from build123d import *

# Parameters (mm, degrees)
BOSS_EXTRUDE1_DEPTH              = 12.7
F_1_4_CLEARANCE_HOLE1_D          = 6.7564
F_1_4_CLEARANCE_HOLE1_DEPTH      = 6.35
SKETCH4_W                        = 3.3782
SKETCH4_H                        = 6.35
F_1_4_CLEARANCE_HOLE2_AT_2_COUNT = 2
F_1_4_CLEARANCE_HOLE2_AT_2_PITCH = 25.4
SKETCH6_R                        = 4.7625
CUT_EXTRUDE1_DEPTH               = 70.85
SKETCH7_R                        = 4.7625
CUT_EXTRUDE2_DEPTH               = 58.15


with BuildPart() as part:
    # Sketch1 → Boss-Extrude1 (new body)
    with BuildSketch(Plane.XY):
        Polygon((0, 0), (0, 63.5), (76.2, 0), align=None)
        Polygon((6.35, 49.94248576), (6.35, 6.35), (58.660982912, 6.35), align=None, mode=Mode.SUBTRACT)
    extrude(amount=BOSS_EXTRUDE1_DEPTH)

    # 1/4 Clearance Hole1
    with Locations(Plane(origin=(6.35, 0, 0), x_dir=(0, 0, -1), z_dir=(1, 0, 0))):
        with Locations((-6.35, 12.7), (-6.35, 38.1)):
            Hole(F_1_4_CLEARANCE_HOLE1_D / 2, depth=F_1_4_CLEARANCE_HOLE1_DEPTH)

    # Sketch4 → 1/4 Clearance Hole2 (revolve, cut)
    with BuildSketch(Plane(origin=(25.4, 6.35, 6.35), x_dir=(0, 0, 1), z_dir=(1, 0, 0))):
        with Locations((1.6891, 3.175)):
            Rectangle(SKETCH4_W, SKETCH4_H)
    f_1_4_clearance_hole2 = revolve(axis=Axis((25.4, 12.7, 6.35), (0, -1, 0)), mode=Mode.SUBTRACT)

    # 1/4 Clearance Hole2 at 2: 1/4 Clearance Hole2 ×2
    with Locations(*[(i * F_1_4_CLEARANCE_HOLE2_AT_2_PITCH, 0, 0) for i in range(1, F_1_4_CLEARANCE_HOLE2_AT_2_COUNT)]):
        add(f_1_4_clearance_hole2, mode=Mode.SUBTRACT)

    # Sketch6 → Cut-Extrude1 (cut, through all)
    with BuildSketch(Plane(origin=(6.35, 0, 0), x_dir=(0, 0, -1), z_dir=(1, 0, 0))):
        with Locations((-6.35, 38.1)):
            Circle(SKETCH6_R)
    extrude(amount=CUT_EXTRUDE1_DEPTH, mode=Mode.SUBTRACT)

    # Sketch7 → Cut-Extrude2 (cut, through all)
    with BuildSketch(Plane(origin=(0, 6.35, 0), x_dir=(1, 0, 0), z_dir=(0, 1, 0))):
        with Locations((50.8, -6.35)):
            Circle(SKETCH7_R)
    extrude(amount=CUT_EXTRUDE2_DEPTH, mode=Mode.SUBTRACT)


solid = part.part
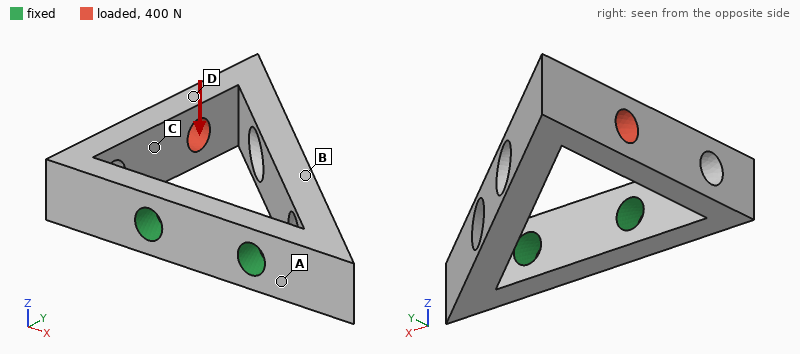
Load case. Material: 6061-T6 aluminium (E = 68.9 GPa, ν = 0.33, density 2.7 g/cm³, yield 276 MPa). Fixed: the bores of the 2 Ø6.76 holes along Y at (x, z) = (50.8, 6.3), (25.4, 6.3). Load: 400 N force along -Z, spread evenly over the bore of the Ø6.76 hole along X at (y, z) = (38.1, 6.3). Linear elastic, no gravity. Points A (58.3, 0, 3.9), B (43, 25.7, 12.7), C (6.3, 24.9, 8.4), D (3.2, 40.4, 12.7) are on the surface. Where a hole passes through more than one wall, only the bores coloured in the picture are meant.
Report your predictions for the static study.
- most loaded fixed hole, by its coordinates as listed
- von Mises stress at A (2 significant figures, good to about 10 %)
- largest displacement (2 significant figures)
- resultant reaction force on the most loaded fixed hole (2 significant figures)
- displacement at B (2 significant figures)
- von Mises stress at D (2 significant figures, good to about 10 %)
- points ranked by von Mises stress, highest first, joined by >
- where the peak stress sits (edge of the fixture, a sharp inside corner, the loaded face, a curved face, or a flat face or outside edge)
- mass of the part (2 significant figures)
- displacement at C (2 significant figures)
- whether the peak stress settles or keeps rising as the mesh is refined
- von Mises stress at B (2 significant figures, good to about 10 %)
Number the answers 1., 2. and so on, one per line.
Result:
1. (25.4, 6.3)
2. 51 MPa
3. 0.52 mm
4. 360 N
5. 0.12 mm
6. 21 MPa
7. A > B > D > C
8. edge of the fixture
9. 38 g
10. 0.19 mm
11. keeps rising
12. 31 MPa
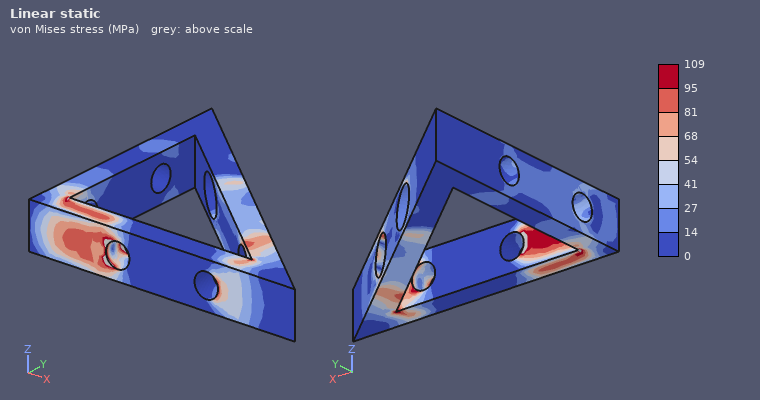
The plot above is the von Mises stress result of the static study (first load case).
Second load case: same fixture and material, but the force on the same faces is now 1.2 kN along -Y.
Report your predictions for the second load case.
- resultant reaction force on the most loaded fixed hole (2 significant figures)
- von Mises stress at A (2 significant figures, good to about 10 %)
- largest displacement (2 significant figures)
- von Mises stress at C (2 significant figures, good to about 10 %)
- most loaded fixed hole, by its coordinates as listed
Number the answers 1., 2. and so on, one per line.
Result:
1. 1.3 kN
2. 22 MPa
3. 0.20 mm
4. 42 MPa
5. (25.4, 6.3)
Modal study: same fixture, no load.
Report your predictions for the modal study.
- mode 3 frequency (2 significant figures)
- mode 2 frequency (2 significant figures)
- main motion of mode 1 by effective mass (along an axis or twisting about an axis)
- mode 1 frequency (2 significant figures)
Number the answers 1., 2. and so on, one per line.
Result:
1. 5100 Hz
2. 2400 Hz
3. along Z
4. 1300 Hz
